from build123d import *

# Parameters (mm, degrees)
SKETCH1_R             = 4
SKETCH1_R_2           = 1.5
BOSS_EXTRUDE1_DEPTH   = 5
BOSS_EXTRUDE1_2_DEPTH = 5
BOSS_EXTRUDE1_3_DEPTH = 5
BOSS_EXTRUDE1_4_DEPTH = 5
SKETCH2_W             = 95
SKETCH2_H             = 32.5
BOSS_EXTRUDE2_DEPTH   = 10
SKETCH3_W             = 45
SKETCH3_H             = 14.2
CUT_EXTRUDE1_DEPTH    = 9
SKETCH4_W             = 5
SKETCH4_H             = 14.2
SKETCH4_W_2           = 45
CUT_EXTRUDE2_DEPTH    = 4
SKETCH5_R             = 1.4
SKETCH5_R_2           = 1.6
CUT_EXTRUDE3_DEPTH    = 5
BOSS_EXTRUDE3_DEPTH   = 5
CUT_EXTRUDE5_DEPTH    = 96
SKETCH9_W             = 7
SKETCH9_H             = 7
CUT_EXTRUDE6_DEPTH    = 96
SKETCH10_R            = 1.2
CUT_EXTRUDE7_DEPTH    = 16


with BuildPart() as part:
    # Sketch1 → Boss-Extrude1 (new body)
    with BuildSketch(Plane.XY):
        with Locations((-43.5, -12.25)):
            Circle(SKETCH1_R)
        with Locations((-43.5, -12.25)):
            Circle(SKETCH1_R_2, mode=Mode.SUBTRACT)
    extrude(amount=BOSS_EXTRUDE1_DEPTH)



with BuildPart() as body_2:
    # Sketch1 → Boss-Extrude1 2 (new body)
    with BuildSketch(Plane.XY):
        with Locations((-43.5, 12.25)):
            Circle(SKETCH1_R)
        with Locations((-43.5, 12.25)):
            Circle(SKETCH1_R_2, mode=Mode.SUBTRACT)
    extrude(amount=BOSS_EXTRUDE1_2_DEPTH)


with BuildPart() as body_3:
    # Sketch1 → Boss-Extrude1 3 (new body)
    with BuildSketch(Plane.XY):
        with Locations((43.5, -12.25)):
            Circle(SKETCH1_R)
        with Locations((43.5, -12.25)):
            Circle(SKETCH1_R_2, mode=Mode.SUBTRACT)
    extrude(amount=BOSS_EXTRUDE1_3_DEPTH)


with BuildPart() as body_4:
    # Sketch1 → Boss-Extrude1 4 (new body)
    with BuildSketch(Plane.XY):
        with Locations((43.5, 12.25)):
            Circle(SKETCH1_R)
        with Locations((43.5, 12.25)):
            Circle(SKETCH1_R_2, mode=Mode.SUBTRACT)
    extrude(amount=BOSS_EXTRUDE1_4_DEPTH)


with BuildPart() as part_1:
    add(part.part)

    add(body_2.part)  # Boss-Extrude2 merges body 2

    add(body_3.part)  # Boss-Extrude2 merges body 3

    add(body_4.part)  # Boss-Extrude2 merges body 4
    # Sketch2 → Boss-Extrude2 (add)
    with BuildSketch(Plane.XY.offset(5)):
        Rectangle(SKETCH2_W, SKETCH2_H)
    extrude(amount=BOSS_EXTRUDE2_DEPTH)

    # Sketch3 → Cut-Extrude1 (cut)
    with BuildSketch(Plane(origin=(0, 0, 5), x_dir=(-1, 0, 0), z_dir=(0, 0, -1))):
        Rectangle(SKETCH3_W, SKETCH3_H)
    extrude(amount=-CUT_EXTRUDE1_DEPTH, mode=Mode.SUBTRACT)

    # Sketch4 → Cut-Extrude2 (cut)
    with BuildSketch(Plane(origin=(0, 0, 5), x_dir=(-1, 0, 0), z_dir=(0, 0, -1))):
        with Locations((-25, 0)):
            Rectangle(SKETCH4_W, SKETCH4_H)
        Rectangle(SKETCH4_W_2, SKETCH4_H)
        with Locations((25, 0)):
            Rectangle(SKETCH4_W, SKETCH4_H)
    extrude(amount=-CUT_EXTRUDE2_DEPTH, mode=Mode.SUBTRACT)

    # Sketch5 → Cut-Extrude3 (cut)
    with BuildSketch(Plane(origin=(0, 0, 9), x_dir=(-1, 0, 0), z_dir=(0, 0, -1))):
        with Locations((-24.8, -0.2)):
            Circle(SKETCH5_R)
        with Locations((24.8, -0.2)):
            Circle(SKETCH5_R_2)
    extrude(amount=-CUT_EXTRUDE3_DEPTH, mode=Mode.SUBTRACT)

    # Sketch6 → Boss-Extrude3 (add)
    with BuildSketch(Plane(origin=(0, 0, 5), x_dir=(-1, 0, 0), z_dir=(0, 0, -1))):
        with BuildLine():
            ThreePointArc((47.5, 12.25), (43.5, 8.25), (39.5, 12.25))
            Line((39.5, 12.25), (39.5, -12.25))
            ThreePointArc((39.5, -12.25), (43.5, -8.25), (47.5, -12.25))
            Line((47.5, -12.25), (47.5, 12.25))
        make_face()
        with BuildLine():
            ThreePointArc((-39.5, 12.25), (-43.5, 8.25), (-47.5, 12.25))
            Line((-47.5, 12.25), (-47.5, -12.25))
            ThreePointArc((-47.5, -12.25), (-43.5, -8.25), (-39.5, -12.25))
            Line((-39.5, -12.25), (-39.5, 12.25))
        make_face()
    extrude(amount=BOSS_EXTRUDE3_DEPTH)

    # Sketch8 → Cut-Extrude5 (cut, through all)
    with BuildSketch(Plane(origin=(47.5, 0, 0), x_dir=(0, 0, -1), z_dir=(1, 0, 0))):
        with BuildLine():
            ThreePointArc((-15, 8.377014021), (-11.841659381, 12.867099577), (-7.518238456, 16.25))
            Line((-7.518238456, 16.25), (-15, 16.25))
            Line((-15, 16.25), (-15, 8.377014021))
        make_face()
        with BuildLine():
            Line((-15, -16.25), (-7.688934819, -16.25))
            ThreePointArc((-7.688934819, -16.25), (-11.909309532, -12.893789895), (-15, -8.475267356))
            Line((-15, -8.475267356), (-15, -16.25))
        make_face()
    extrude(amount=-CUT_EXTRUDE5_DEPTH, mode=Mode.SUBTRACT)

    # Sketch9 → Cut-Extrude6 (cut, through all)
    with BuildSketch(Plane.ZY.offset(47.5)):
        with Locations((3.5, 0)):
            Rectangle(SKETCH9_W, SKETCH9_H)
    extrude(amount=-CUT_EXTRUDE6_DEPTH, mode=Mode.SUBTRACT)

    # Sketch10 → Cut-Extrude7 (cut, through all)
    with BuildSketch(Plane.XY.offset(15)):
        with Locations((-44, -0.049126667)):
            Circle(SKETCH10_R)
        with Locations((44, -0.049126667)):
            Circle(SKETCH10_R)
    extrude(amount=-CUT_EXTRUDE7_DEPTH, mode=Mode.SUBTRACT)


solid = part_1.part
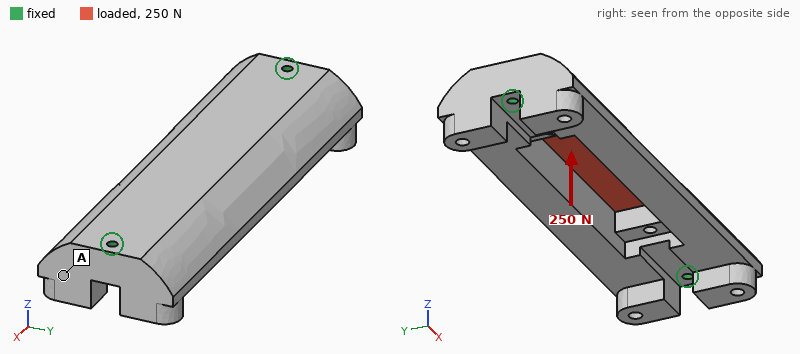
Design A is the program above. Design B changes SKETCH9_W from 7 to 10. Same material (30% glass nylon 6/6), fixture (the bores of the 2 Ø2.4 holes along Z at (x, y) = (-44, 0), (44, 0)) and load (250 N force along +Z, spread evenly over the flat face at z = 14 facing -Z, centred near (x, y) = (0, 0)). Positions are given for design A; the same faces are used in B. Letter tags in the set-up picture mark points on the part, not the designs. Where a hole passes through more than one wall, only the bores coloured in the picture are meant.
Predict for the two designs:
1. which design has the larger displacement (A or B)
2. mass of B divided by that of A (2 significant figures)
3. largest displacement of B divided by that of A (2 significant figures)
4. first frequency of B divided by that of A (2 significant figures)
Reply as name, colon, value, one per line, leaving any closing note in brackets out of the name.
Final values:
which design has the larger displacement: B
mass of B divided by that of A: 0.98
largest displacement of B divided by that of A: 1.1
first frequency of B divided by that of A: 0.91
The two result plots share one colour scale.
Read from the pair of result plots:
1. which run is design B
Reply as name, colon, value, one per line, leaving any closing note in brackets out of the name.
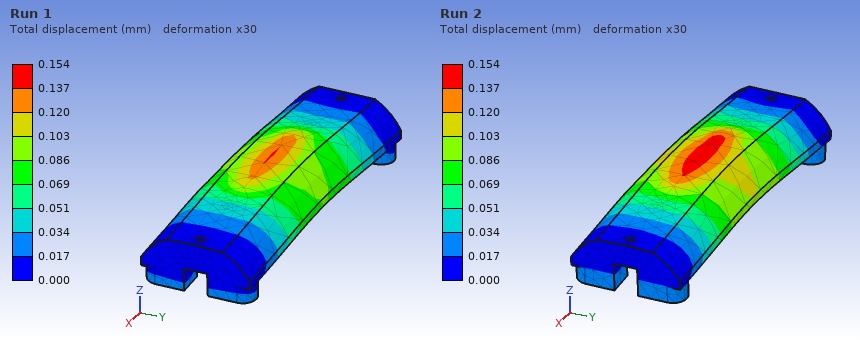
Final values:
which run is design B: Run 2
